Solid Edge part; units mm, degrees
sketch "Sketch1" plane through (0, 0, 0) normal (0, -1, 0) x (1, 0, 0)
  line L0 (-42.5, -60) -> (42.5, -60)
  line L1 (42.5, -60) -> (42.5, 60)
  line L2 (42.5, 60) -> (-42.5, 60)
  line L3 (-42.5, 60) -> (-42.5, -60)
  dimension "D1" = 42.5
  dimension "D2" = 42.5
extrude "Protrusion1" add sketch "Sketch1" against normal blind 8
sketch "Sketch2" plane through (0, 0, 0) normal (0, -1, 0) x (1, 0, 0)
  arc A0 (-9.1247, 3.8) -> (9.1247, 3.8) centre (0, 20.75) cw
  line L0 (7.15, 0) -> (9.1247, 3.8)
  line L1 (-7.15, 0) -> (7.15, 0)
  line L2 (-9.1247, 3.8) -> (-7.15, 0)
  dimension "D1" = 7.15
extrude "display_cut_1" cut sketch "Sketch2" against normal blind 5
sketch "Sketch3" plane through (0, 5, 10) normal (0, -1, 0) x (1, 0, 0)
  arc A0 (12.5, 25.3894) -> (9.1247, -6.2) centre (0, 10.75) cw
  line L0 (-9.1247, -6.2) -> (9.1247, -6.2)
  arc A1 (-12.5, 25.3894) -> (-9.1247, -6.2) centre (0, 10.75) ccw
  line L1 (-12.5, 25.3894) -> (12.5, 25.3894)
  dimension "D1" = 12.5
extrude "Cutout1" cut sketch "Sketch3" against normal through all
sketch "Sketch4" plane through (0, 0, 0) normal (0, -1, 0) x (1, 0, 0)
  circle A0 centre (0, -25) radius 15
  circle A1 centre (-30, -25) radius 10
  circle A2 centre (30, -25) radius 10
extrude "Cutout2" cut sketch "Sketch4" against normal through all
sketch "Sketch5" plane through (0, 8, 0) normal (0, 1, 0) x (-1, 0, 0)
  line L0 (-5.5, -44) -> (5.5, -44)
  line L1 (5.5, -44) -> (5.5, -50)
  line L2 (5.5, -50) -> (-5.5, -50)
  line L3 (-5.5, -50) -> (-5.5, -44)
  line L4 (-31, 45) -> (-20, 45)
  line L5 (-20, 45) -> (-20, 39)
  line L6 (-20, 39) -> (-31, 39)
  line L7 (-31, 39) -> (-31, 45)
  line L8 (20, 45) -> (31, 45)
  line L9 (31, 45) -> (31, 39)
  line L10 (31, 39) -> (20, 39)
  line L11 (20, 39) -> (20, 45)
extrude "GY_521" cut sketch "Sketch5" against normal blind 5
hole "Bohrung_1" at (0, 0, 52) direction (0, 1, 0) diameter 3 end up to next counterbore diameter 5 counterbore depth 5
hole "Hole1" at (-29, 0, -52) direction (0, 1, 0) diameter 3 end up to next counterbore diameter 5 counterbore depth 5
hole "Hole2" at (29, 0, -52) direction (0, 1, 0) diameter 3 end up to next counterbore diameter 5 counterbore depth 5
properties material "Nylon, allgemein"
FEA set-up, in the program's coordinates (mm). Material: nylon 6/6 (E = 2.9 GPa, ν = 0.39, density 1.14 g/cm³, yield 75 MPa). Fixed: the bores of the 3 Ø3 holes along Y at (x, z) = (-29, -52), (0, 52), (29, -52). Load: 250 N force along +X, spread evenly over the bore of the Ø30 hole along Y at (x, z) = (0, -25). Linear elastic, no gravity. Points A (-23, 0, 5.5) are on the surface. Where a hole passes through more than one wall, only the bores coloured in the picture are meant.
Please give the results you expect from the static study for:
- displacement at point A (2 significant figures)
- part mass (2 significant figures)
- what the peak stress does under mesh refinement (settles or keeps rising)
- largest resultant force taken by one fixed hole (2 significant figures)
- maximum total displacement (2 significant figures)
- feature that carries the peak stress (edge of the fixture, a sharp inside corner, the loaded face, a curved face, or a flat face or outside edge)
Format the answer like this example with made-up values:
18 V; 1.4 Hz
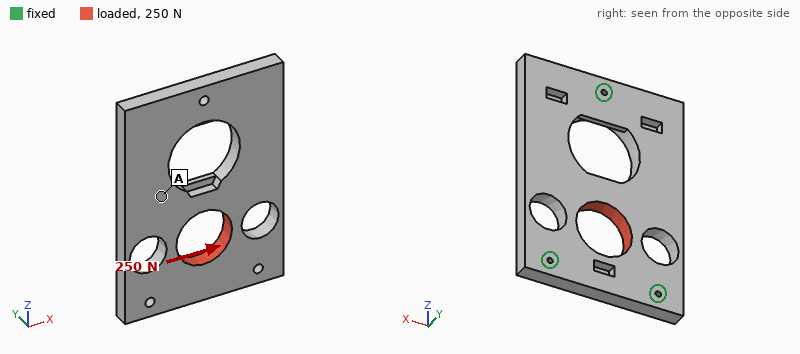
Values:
37 µm; 69 g; keeps rising; 99 N; 43 µm; edge of the fixture
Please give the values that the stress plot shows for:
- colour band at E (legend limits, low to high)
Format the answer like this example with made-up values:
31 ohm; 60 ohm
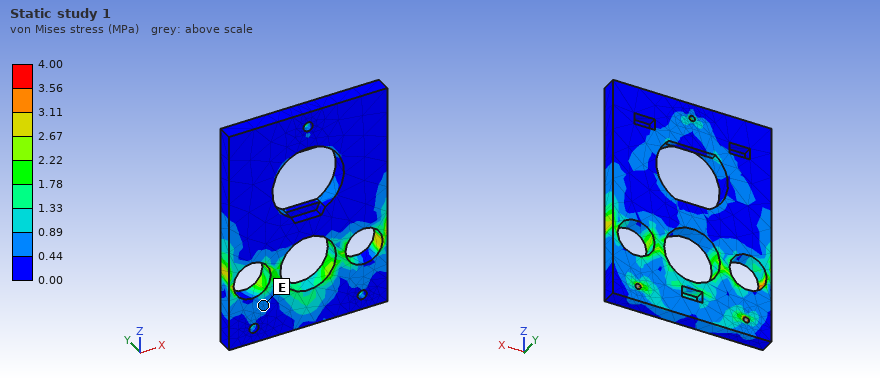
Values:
0.44 to 0.89 MPa
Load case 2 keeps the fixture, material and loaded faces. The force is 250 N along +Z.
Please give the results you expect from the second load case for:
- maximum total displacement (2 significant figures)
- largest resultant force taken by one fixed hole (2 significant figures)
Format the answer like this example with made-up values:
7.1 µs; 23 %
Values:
37 µm; 99 N
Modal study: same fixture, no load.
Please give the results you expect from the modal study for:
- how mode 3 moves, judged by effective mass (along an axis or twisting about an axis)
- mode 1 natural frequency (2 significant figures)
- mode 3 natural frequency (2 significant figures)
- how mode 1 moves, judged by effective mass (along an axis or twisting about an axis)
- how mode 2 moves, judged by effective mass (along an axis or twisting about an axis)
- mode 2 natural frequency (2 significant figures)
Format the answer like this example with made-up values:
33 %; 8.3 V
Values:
twisting about X; 440 Hz; 1200 Hz; twisting about Z; along Y; 590 Hz
